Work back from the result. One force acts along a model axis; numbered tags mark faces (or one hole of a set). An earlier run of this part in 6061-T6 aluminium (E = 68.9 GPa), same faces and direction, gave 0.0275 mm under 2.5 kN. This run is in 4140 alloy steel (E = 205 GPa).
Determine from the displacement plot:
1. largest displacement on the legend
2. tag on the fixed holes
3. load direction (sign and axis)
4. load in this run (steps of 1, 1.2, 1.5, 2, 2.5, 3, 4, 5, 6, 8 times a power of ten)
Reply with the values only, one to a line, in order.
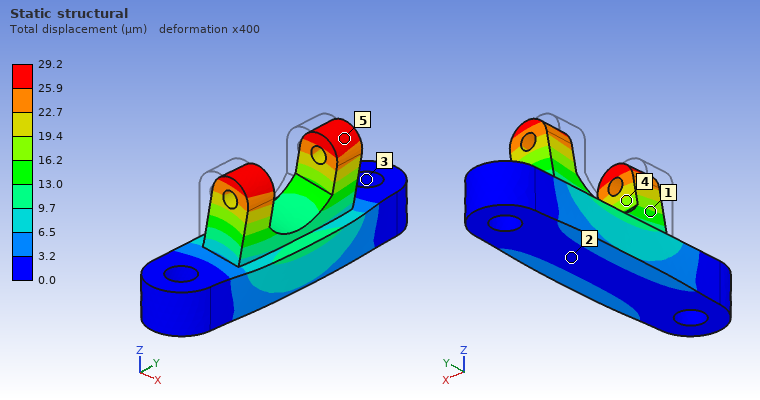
29.2 µm
3
+X
8 kN
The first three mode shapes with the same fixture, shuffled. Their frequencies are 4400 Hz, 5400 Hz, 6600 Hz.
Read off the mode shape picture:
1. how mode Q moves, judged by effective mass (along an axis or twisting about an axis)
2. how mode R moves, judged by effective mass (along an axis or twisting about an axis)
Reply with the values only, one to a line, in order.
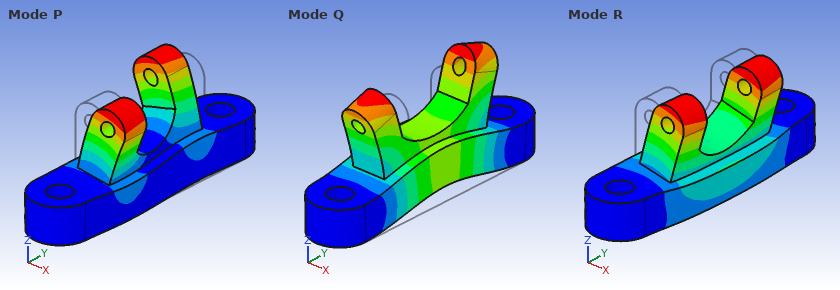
along Z
along X
